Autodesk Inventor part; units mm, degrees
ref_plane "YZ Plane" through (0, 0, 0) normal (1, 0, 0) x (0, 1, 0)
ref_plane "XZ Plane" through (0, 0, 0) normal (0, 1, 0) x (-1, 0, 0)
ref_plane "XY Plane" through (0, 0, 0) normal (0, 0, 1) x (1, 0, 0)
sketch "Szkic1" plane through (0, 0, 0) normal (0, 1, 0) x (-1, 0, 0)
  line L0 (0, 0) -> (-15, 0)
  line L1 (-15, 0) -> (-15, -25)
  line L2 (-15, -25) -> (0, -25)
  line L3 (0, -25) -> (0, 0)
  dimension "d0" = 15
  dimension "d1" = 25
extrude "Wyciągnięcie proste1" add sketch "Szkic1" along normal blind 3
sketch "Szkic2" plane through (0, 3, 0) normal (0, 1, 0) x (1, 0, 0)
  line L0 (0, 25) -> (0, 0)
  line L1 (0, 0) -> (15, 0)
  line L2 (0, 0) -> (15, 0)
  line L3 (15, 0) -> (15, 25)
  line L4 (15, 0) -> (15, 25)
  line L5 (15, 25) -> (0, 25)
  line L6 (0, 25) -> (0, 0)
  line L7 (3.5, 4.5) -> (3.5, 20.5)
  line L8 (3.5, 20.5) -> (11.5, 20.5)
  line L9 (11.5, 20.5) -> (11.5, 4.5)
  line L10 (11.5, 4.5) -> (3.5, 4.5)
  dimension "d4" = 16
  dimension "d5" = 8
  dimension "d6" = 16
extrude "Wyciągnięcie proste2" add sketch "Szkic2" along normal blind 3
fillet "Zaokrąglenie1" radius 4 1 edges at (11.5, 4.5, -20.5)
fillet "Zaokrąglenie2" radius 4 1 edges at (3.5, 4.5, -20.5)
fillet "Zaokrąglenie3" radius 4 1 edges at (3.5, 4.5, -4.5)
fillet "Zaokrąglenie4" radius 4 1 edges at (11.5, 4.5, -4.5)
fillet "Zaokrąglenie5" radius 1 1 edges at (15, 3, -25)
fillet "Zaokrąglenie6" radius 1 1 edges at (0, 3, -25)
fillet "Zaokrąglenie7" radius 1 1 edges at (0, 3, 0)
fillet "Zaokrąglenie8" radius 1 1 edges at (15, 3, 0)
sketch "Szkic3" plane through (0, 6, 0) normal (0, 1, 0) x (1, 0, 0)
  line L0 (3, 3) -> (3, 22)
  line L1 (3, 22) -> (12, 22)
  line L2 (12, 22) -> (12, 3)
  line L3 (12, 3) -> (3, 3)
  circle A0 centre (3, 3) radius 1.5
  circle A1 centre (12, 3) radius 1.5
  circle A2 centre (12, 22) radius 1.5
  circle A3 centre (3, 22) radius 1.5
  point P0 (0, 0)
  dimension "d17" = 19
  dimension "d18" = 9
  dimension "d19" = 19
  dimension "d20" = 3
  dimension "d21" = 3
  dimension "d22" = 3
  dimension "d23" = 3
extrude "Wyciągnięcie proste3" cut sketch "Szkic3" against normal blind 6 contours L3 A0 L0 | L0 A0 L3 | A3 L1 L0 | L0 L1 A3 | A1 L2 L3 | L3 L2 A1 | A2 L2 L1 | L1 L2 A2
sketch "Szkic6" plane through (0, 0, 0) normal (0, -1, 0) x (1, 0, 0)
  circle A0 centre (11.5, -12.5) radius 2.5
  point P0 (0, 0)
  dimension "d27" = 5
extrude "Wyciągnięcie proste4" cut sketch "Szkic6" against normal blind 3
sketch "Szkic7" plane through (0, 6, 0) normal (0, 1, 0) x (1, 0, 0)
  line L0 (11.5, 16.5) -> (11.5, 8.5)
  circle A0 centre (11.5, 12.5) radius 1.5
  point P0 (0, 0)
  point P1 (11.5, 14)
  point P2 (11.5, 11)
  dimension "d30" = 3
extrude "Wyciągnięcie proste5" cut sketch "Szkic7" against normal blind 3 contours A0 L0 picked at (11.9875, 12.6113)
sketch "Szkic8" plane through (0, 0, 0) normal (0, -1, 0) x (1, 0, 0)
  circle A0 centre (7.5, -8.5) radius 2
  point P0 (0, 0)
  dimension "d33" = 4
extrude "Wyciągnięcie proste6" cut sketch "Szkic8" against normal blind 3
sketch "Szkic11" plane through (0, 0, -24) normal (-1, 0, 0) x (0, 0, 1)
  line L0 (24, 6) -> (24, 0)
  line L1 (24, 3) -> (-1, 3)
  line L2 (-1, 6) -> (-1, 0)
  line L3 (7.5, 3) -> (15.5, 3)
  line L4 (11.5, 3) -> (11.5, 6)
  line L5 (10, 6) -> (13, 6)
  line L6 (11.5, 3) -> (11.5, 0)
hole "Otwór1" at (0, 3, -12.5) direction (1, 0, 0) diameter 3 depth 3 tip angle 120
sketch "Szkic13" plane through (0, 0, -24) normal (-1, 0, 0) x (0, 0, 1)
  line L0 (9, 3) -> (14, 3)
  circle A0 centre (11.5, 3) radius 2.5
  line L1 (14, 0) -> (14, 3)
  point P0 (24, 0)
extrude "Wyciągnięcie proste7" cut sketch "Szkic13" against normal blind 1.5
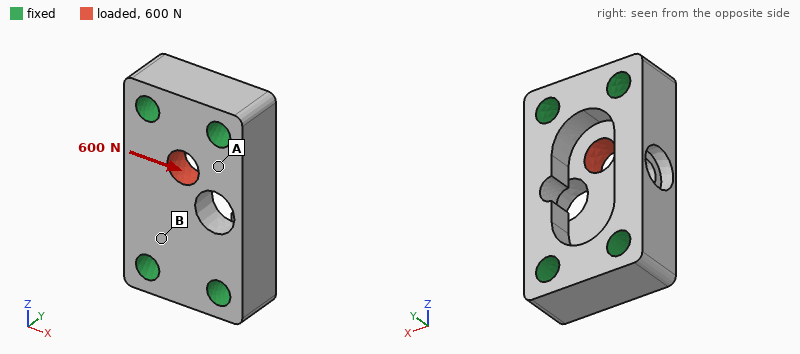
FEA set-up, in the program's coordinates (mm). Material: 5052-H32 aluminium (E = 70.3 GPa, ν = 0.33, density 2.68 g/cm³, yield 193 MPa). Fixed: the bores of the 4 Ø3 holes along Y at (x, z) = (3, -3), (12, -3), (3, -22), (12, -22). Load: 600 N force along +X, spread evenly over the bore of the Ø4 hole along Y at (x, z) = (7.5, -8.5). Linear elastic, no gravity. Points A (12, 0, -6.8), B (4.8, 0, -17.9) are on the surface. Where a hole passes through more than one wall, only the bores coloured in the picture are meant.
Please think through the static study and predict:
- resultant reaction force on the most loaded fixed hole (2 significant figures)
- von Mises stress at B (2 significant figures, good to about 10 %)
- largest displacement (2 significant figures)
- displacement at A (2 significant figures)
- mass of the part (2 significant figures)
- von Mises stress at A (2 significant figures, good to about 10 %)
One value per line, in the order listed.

250 N
5.5 MPa
3.2 µm
1.2 µm
4.2 g
15 MPa
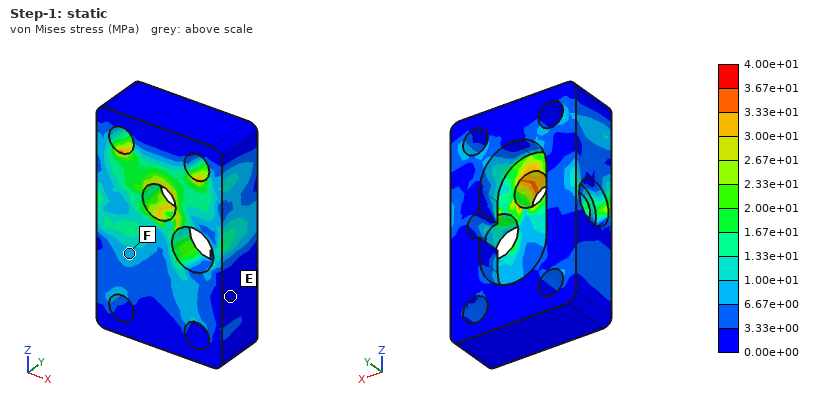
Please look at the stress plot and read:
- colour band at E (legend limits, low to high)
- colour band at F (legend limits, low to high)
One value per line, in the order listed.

0.00e+00 to 3.33e+00 MPa
6.67e+00 to 1.00e+01 MPa
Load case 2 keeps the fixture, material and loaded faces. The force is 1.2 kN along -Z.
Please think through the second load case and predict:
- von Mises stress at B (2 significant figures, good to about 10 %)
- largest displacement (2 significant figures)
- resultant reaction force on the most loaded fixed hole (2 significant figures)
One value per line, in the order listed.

12 MPa
3.8 µm
470 N
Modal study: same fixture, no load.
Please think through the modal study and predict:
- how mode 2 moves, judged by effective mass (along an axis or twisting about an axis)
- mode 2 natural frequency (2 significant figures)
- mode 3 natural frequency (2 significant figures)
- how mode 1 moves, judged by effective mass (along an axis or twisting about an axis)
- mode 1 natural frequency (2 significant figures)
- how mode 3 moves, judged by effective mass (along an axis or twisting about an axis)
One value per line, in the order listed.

along X
73 kHz
80 kHz
along Y
66 kHz
along X
